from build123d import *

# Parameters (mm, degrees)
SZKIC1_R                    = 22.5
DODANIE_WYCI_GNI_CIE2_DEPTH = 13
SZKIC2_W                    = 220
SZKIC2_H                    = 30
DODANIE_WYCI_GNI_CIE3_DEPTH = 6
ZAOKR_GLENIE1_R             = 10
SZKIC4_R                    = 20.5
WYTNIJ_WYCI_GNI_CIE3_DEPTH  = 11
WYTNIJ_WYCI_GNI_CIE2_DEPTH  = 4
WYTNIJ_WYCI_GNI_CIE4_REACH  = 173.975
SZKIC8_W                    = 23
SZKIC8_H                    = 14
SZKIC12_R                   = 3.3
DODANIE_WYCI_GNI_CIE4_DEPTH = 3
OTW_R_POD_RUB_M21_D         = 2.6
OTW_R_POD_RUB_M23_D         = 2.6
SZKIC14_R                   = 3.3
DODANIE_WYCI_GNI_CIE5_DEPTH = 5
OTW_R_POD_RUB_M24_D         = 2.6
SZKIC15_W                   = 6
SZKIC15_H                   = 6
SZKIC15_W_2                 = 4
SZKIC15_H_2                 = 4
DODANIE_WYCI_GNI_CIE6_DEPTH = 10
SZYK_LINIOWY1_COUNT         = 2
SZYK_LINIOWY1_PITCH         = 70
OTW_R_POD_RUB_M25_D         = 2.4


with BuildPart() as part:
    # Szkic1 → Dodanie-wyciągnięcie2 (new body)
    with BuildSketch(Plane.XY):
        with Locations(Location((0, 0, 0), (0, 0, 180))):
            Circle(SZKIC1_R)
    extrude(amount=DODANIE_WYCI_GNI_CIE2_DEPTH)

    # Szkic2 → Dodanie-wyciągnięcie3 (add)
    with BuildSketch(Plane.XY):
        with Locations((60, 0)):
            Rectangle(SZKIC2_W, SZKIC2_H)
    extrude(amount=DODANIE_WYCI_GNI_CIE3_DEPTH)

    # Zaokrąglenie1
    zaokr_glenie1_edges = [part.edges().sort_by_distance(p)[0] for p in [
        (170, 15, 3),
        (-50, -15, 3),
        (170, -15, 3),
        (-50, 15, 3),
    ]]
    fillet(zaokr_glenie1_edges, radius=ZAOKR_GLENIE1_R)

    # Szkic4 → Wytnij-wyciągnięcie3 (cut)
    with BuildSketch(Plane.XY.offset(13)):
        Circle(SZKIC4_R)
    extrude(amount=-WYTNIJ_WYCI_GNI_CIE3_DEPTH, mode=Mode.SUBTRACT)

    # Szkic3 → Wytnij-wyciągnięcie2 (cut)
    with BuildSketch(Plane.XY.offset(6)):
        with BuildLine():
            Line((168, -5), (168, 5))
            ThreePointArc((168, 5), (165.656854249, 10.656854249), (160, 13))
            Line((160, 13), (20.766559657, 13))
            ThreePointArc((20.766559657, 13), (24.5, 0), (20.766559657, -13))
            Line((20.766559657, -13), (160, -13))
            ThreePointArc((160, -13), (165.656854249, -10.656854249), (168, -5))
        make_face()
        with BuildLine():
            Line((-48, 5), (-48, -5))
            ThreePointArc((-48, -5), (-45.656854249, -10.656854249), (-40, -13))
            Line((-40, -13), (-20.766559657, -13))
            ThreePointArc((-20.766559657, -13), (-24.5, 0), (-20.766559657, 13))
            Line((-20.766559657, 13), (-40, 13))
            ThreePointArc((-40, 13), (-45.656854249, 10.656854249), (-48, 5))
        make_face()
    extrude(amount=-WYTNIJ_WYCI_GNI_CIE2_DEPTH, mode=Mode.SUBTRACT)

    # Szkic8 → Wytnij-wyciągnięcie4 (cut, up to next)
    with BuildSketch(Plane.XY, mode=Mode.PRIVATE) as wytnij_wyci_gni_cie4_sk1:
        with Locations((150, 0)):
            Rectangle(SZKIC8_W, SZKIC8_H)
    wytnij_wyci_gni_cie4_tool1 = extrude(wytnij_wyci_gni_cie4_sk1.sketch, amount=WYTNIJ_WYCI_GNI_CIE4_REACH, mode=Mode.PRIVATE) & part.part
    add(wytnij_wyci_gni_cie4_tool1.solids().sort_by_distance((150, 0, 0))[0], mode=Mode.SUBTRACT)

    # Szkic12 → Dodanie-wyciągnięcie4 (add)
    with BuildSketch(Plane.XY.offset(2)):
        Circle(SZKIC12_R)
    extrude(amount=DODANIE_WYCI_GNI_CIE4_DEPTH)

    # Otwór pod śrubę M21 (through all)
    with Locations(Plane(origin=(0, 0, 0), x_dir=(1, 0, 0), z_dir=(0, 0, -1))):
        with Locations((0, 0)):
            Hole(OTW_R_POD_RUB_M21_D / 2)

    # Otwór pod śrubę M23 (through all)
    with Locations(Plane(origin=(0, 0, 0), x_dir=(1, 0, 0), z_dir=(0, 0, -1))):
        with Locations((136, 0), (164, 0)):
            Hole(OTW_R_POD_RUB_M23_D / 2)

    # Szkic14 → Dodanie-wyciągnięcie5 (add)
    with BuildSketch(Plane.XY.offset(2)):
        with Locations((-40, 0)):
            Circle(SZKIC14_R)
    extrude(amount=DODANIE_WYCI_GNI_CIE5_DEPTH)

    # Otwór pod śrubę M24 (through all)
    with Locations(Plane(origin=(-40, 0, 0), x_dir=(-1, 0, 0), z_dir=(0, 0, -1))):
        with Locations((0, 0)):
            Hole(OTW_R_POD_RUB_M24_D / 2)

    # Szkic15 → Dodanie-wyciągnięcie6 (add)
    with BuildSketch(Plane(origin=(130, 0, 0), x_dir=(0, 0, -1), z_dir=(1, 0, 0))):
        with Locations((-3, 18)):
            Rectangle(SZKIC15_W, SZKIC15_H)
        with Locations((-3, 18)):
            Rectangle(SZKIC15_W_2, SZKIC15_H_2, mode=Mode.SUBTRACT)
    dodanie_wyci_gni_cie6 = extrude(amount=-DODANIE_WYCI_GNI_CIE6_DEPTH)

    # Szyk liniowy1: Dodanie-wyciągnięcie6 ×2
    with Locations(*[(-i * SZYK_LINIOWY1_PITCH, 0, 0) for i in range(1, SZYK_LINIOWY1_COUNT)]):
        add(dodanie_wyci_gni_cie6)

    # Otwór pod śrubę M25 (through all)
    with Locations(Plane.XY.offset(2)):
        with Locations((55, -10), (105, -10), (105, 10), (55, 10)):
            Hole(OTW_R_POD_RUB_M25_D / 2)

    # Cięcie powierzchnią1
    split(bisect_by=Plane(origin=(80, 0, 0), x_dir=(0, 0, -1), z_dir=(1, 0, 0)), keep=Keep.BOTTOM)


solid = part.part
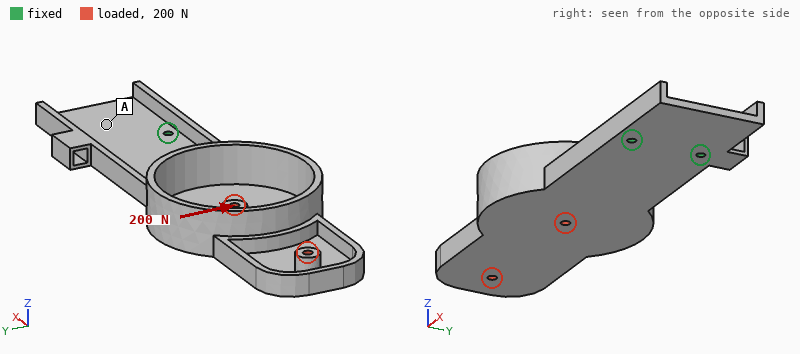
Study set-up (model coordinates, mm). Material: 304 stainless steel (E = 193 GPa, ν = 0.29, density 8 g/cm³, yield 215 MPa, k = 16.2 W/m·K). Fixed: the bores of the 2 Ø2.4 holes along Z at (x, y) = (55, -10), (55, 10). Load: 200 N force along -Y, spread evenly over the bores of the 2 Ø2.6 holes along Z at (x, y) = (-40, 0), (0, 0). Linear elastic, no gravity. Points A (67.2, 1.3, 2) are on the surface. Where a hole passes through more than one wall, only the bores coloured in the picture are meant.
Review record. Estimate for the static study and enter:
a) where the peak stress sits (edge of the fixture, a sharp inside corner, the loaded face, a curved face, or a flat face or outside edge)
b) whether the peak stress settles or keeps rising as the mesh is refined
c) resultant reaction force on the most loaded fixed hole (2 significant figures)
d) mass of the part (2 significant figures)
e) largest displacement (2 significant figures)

edge of the fixture
keeps rising
760 N
110 g
54 µm
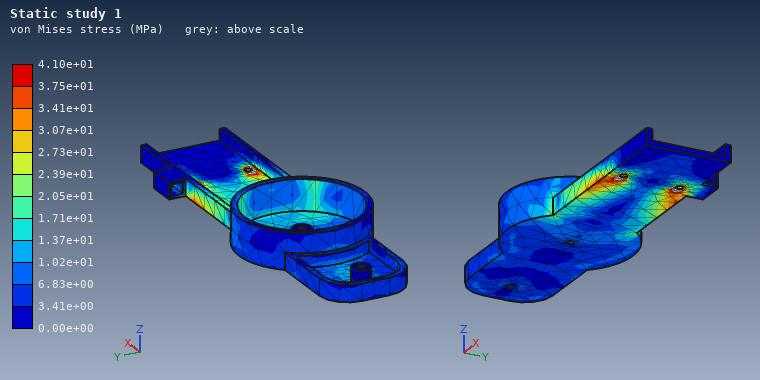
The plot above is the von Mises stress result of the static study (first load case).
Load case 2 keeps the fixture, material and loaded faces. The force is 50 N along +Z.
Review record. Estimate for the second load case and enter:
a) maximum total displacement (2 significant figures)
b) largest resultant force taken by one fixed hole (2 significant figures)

0.57 mm
37 N
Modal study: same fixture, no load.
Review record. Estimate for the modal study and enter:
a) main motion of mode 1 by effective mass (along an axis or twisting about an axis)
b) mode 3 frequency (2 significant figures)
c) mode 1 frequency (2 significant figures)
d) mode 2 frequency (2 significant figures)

along Z
1700 Hz
250 Hz
980 Hz
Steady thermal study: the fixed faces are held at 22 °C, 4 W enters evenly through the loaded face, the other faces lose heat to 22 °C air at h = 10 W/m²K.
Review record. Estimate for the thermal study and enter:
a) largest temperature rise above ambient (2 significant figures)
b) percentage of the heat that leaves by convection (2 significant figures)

78 K
86 %
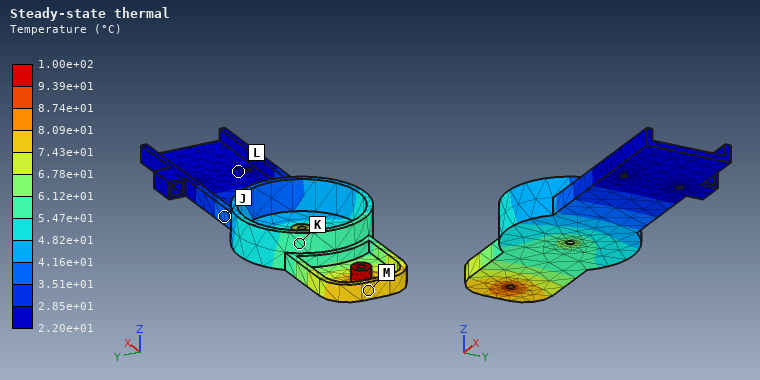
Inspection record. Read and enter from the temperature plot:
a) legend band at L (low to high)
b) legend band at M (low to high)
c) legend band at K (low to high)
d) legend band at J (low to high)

2.20e+01 to 2.85e+01 °C
7.43e+01 to 8.09e+01 °C
5.47e+01 to 6.12e+01 °C
3.51e+01 to 4.16e+01 °C
